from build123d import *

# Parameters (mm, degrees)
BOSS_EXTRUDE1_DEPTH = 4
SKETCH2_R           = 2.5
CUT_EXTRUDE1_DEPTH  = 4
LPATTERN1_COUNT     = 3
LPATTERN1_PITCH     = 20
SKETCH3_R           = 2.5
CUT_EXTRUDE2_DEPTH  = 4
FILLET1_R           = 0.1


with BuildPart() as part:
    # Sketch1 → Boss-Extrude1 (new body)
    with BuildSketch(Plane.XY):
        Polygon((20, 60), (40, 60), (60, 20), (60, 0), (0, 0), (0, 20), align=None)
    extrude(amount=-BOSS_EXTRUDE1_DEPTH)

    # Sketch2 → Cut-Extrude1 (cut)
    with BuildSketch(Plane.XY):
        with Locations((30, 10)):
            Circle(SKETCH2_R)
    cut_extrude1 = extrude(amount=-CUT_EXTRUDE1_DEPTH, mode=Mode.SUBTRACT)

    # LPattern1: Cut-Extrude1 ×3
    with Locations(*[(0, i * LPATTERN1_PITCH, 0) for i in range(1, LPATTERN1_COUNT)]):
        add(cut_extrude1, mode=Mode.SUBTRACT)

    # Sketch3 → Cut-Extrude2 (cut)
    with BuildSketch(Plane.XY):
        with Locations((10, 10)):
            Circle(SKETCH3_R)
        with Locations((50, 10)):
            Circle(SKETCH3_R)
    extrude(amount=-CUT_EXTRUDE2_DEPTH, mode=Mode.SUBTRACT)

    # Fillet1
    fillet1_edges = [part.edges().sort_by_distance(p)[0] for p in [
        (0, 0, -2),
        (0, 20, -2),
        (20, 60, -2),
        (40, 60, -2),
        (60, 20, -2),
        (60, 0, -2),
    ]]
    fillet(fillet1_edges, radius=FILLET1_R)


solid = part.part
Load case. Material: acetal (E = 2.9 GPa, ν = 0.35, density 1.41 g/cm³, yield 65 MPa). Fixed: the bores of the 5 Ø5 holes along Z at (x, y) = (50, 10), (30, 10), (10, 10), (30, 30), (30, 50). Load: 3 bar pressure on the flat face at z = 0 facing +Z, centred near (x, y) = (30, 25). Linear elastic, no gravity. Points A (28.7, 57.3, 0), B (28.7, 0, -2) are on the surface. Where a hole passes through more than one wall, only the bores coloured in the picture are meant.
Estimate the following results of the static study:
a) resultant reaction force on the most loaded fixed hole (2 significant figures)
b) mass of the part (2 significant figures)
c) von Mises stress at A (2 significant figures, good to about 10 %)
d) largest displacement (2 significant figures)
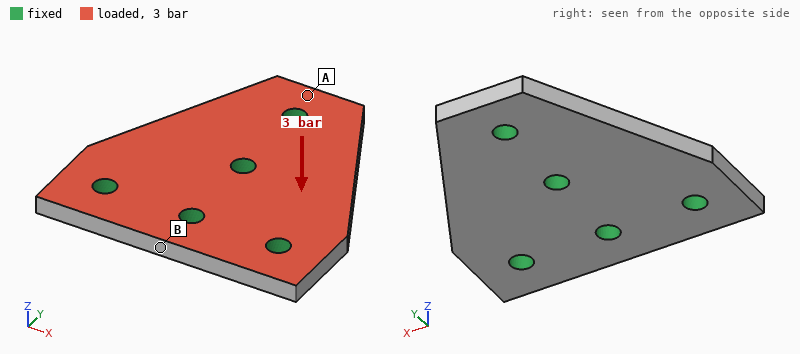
200 N
15 g
6.0 MPa
0.22 mm
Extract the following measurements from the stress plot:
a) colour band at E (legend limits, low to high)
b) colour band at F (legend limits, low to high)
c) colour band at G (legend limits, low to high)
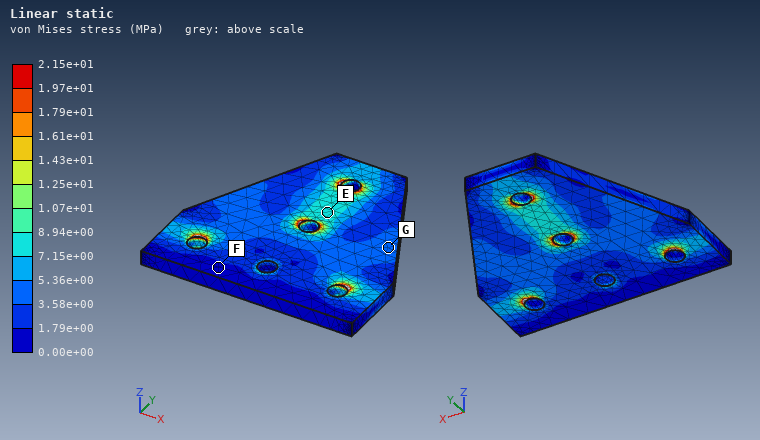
7.15e+00 to 8.94e+00 MPa
0.00e+00 to 1.79e+00 MPa
3.58e+00 to 5.36e+00 MPa
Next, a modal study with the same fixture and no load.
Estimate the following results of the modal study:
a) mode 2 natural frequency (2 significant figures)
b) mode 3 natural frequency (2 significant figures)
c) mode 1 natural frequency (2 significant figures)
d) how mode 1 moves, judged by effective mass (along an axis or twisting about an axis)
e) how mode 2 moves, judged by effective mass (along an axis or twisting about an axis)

3400 Hz
5700 Hz
3200 Hz
twisting about Y
along Z
